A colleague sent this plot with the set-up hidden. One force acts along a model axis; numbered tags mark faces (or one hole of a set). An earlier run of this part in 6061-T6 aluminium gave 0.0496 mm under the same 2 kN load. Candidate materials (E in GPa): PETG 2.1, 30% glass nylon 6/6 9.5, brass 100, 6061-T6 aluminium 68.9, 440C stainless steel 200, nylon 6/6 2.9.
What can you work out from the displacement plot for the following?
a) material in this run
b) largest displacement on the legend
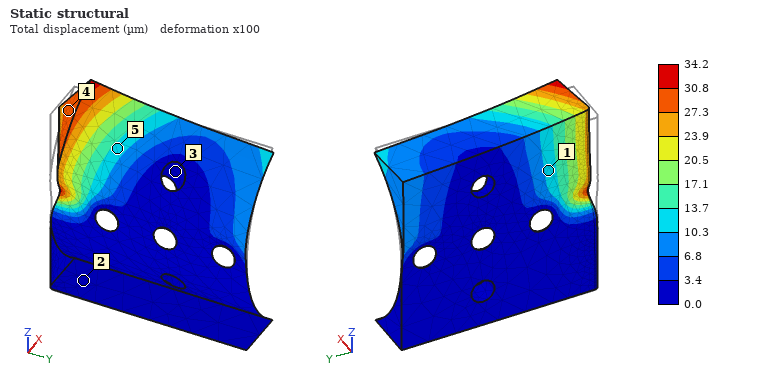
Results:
brass
34.2 µm
